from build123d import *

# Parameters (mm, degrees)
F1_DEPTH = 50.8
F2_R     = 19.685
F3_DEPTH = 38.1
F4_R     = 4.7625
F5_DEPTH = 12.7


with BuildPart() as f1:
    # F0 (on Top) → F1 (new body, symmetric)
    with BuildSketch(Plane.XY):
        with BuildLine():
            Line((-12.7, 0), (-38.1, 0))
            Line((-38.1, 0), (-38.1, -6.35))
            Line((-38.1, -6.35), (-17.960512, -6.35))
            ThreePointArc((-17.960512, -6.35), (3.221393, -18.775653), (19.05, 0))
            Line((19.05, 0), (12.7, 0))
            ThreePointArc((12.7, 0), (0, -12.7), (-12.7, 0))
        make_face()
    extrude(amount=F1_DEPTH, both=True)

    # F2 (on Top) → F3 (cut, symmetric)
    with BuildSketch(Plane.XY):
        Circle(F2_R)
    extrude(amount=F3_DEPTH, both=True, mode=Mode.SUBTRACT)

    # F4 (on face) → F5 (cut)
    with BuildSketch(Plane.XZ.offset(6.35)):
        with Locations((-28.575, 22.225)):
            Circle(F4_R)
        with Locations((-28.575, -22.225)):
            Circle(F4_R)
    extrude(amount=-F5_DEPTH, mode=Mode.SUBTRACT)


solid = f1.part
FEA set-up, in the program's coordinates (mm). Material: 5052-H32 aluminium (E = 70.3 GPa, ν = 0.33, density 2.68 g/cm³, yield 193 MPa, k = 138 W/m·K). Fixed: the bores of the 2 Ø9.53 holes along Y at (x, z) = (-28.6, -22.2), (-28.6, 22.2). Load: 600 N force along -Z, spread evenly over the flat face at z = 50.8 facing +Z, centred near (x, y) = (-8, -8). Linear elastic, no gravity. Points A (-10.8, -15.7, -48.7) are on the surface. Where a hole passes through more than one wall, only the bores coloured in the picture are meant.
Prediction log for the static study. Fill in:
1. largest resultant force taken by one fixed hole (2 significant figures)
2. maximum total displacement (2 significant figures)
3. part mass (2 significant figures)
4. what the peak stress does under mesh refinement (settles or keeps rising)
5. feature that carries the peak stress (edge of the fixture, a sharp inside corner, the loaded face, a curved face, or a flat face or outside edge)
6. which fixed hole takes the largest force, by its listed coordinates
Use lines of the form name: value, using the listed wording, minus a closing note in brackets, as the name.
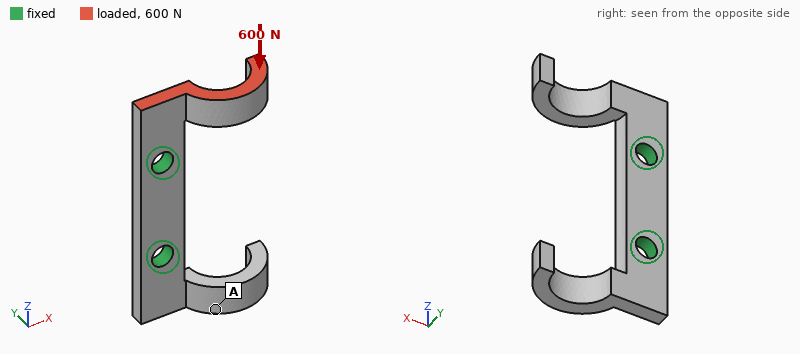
largest resultant force taken by one fixed hole: 600 N
maximum total displacement: 0.20 mm
part mass: 52 g
what the peak stress does under mesh refinement: keeps rising
feature that carries the peak stress: a sharp inside corner
which fixed hole takes the largest force, by its listed coordinates: (-28.6, 22.2)
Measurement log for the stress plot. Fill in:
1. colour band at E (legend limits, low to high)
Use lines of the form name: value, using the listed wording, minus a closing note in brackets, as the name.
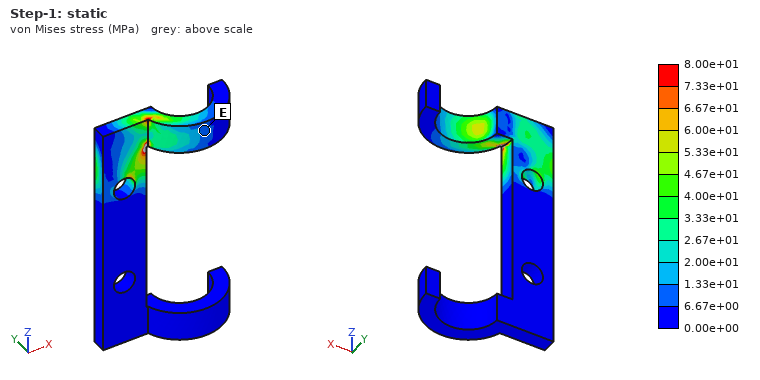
colour band at E: 6.67e+00 to 1.33e+01 MPa
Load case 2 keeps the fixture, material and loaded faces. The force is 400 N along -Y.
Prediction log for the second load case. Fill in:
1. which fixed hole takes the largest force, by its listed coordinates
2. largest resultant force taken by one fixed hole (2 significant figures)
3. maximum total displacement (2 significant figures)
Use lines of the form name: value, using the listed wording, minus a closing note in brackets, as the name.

which fixed hole takes the largest force, by its listed coordinates: (-28.6, 22.2)
largest resultant force taken by one fixed hole: 400 N
maximum total displacement: 0.48 mm
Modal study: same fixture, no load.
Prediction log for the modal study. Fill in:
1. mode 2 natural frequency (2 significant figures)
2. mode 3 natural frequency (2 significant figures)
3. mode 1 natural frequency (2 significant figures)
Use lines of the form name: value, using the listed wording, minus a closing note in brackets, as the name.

mode 2 natural frequency: 1500 Hz
mode 3 natural frequency: 2700 Hz
mode 1 natural frequency: 1500 Hz
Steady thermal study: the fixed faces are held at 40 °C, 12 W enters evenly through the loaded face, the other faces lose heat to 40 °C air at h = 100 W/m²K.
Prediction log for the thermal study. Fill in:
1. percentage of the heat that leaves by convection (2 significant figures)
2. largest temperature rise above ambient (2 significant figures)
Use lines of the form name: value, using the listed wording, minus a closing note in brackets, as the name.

percentage of the heat that leaves by convection: 32 %
largest temperature rise above ambient: 23 K
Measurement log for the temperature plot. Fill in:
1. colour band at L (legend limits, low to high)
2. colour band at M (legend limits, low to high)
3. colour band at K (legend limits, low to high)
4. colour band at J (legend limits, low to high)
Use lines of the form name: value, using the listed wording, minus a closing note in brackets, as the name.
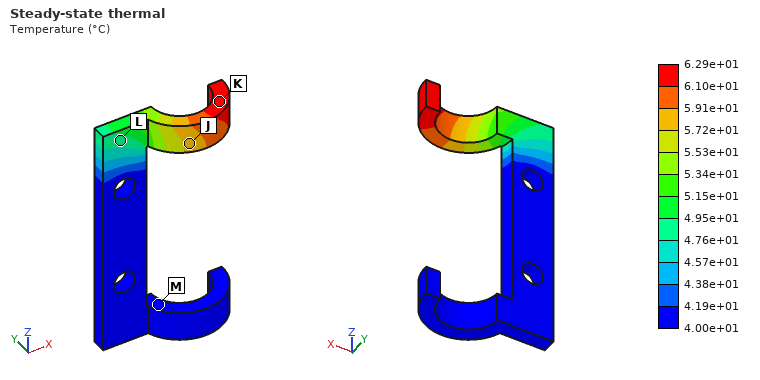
colour band at L: 4.76e+01 to 4.95e+01 °C
colour band at M: 4.00e+01 to 4.19e+01 °C
colour band at K: 6.10e+01 to 6.29e+01 °C
colour band at J: 5.72e+01 to 5.91e+01 °C
